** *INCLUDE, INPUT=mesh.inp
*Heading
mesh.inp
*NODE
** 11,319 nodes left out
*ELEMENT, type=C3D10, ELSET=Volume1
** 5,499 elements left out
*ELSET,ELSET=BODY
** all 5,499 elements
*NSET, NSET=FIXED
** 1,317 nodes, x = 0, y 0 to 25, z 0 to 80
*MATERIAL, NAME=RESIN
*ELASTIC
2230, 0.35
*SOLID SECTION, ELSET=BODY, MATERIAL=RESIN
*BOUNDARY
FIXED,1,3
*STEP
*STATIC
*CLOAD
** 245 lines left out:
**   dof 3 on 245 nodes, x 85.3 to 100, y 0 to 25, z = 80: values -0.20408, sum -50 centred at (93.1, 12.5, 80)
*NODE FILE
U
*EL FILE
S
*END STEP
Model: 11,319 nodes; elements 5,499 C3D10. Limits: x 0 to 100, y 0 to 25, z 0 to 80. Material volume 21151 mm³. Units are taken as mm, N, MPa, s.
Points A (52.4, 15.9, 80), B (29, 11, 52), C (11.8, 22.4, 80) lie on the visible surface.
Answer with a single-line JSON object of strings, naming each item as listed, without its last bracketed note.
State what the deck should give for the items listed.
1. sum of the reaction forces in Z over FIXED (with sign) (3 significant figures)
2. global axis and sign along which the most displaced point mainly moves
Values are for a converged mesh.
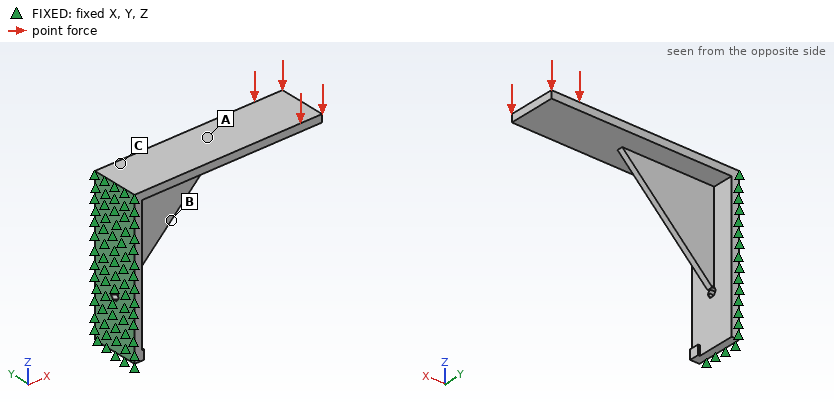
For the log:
{"sum of the reaction forces in Z over FIXED (with sign)": "50.0 N", "global axis and sign along which the most displaced point mainly moves": "-Z"}
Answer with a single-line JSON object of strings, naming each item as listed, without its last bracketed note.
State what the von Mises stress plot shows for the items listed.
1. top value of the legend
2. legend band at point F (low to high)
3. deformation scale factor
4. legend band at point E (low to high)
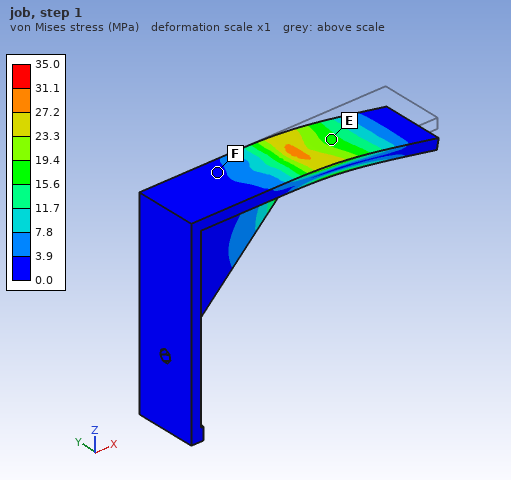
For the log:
{"top value of the legend": "35.0 MPa", "legend band at point F": "0.0 to 3.9 MPa", "deformation scale factor": "1", "legend band at point E": "15.6 to 19.4 MPa"}
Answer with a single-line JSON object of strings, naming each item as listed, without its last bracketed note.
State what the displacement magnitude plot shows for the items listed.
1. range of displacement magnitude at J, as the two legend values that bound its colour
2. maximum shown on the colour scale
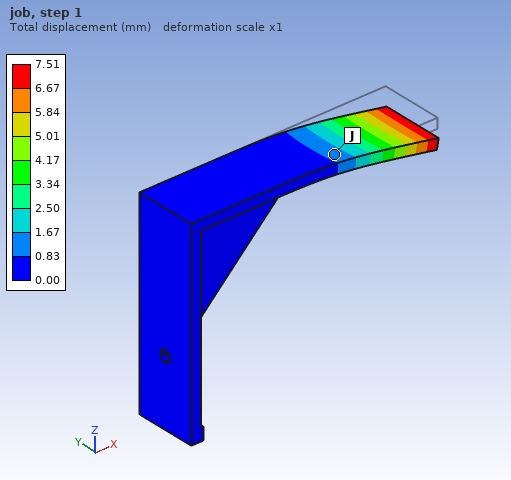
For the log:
{"range of displacement magnitude at J, as the two legend values that bound its colour": "0.83 to 1.67 mm", "maximum shown on the colour scale": "7.51 mm"}
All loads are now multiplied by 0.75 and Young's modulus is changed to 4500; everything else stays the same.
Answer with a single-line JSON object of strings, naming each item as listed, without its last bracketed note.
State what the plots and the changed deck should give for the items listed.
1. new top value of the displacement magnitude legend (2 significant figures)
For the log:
{"new top value of the displacement magnitude legend": "2.8 mm"}
